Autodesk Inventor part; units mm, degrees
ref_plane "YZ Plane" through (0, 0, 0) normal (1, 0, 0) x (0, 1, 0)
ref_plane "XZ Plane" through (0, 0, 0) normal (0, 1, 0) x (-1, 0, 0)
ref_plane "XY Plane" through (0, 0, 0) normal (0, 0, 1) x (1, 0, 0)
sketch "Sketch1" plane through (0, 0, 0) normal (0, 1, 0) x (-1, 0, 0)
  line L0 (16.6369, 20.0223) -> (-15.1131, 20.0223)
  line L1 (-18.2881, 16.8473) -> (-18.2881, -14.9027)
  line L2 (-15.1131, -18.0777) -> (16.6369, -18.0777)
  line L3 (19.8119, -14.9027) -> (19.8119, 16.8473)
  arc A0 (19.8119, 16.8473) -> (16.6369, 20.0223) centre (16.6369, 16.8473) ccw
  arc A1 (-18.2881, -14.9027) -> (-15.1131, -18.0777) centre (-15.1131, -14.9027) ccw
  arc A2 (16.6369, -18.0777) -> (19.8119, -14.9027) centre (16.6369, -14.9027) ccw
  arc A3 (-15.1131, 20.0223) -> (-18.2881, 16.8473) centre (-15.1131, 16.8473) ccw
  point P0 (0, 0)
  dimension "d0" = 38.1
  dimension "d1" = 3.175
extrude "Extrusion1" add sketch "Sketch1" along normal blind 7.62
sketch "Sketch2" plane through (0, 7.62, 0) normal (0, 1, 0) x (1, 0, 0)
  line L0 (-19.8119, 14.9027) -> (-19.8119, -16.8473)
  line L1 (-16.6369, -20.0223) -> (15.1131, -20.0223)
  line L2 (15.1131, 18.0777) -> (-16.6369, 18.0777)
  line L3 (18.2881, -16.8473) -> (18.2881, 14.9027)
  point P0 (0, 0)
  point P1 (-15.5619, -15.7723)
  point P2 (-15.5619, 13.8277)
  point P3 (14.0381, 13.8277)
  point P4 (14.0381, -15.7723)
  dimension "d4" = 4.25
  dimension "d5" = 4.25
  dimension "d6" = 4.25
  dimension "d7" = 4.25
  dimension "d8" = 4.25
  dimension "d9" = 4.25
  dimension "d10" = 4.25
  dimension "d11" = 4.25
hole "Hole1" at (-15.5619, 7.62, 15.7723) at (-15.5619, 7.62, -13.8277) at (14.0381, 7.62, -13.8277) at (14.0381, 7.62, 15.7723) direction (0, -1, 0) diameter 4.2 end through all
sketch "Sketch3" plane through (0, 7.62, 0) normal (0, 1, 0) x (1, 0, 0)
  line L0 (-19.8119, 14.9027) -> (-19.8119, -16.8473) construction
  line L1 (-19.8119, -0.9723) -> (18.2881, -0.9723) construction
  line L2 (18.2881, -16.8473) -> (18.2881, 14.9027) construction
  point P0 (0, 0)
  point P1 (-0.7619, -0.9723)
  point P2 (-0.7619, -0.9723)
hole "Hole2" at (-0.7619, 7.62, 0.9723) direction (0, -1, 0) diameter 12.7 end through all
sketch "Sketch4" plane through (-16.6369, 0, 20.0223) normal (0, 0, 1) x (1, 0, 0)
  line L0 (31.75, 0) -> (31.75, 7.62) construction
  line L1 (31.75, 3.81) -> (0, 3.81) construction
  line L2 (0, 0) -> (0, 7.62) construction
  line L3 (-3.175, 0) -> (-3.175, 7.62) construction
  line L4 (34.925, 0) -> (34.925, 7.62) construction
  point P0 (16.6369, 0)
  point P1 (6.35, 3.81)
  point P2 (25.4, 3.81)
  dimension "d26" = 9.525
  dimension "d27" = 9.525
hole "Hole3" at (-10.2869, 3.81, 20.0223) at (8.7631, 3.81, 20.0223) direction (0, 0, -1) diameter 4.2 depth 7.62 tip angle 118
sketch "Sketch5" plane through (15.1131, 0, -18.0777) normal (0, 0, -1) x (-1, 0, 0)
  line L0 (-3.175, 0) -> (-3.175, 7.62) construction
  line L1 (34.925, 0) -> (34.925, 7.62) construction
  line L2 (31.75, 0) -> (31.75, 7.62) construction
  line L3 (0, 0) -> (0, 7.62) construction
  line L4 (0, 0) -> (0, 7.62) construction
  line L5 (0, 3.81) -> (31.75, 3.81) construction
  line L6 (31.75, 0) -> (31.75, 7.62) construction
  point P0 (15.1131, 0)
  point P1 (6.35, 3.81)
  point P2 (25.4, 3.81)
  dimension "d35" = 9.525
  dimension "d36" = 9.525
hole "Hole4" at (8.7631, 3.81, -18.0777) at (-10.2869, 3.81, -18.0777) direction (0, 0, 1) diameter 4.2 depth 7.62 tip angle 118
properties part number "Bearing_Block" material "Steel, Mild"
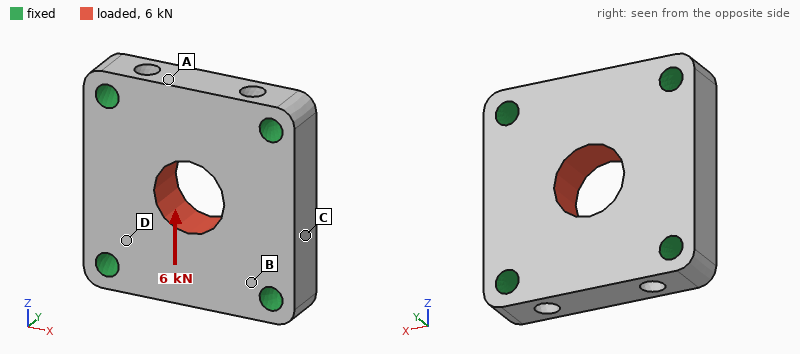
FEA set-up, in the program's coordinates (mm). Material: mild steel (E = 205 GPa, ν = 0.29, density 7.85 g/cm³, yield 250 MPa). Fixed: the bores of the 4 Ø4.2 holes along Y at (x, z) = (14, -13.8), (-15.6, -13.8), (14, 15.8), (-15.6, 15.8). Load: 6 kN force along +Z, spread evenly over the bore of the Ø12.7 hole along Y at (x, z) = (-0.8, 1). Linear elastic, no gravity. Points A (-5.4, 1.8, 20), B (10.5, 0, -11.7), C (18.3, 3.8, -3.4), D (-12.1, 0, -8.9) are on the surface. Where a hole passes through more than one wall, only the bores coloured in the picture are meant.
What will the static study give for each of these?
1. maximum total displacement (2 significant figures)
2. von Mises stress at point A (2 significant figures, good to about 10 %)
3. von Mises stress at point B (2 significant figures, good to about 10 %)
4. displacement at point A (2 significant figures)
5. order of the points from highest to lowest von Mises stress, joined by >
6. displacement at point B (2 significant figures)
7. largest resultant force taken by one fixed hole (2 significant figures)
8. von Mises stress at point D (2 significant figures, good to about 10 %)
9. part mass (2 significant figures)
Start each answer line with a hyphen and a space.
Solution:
- 2.5 µm
- 13 MPa
- 32 MPa
- 1.7 µm
- B > D > A > C
- 0.55 µm
- 1.6 kN
- 27 MPa
- 72 g
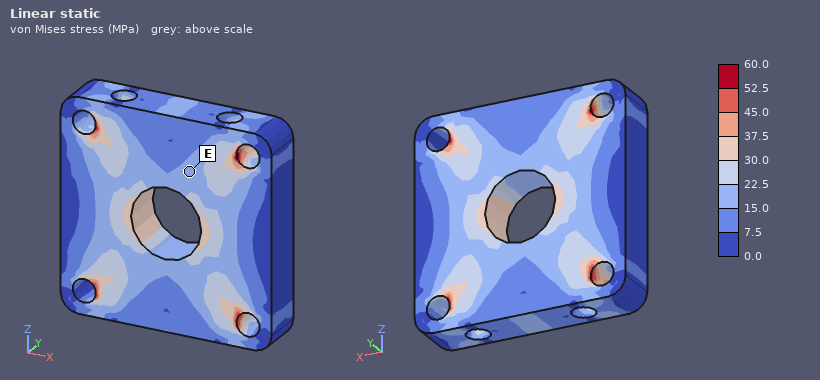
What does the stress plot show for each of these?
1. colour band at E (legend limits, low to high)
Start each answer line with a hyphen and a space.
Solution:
- 15.0 to 22.5 MPa
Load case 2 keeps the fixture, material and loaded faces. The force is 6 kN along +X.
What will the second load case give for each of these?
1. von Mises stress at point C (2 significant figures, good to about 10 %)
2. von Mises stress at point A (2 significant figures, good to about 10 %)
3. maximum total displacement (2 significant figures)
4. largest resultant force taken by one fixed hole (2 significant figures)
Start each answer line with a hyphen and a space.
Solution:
- 15 MPa
- 5.7 MPa
- 2.4 µm
- 1.6 kN
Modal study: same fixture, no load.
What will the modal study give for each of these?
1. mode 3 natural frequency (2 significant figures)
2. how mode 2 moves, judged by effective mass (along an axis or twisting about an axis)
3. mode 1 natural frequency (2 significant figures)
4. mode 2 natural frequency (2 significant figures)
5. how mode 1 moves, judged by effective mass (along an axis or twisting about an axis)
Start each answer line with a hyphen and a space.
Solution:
- 35 kHz
- twisting about X
- 25 kHz
- 30 kHz
- along Y
